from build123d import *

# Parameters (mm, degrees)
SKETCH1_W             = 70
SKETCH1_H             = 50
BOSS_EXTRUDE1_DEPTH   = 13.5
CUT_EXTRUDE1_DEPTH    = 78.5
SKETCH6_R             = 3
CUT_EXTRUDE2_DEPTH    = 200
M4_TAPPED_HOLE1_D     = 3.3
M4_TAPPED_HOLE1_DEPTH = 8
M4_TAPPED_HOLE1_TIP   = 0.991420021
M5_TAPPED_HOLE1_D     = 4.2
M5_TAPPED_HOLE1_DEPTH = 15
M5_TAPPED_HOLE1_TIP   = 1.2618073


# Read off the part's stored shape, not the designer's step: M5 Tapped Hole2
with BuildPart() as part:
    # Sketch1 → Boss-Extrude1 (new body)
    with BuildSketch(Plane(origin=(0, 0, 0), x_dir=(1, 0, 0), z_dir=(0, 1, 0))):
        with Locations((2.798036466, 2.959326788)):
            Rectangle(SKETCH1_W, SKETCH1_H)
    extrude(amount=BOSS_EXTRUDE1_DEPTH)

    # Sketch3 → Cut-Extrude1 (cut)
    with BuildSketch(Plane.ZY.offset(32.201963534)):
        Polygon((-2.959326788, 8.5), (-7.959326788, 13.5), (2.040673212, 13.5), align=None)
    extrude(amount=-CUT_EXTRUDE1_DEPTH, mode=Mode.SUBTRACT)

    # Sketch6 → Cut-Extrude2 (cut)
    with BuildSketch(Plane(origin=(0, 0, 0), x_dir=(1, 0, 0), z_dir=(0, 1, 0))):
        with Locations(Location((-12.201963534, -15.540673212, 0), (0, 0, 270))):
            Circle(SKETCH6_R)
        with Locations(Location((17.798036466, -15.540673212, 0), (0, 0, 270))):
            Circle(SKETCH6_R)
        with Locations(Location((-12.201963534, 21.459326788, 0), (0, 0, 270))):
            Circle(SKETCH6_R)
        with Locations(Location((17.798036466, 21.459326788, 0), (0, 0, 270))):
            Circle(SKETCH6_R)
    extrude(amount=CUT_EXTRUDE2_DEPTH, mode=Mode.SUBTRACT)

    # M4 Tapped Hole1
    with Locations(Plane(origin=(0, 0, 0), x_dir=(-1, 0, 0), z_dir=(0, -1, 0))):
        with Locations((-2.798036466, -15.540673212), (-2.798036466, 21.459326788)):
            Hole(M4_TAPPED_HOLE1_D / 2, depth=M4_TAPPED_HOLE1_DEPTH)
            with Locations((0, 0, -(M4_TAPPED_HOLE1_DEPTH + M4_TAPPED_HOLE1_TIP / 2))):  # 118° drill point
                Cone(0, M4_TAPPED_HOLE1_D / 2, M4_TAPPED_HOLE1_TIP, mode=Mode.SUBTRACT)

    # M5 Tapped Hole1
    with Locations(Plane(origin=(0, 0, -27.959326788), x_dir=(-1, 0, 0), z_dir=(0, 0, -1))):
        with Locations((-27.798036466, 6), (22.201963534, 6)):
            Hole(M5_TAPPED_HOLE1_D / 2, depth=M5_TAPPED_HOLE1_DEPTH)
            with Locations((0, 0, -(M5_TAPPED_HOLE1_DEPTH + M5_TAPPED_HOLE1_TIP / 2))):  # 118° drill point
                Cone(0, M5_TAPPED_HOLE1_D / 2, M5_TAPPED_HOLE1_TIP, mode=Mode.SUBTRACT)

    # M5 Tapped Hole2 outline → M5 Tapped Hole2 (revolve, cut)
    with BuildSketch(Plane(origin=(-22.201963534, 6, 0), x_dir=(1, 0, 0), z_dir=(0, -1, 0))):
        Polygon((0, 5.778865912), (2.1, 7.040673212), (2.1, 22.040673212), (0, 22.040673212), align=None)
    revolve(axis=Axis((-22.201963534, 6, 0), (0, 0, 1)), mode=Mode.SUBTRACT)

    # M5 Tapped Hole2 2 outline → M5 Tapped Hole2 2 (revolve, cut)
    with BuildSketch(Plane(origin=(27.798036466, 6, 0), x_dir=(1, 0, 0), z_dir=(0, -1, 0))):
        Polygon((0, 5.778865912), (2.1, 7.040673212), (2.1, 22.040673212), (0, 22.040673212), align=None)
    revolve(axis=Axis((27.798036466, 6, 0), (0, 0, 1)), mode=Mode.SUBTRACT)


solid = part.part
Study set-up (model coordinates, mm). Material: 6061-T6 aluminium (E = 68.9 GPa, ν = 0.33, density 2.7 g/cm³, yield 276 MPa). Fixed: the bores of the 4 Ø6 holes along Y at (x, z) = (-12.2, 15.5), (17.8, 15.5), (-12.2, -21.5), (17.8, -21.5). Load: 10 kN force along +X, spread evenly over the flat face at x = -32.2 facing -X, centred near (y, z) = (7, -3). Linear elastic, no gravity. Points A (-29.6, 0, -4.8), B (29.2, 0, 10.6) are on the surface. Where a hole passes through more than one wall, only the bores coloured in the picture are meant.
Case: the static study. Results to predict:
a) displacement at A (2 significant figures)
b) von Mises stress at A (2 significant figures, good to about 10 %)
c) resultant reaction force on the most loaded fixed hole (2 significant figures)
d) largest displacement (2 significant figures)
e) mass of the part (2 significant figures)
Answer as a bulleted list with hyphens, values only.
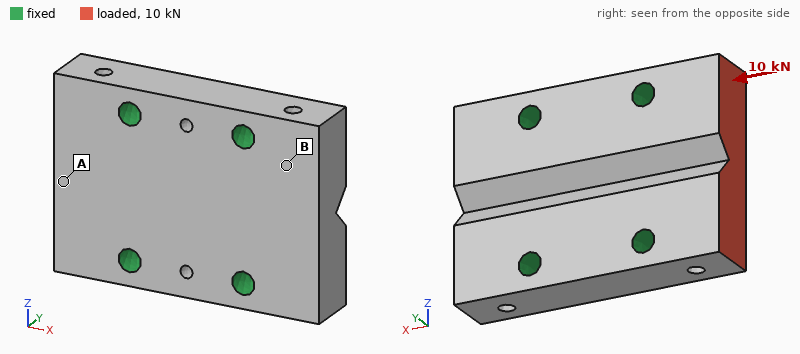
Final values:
- 6.2 µm
- 14 MPa
- 4.3 kN
- 6.8 µm
- 120 g
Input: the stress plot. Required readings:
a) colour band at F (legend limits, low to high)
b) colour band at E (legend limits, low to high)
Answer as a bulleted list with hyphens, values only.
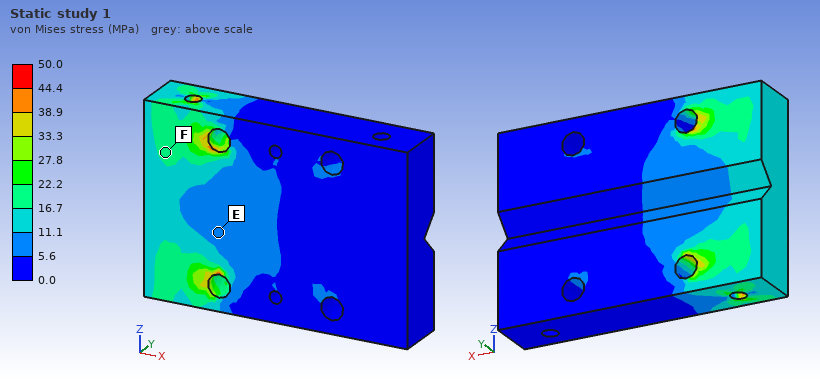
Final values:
- 16.7 to 22.2 MPa
- 5.6 to 11.1 MPa
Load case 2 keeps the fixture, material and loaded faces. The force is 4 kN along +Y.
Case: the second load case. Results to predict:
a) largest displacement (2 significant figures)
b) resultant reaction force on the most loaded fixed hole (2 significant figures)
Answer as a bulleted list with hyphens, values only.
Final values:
- 31 µm
- 2.3 kN
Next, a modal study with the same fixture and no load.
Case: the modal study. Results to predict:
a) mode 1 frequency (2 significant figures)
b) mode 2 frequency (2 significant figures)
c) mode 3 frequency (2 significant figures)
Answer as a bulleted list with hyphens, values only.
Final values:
- 18 kHz
- 18 kHz
- 26 kHz
